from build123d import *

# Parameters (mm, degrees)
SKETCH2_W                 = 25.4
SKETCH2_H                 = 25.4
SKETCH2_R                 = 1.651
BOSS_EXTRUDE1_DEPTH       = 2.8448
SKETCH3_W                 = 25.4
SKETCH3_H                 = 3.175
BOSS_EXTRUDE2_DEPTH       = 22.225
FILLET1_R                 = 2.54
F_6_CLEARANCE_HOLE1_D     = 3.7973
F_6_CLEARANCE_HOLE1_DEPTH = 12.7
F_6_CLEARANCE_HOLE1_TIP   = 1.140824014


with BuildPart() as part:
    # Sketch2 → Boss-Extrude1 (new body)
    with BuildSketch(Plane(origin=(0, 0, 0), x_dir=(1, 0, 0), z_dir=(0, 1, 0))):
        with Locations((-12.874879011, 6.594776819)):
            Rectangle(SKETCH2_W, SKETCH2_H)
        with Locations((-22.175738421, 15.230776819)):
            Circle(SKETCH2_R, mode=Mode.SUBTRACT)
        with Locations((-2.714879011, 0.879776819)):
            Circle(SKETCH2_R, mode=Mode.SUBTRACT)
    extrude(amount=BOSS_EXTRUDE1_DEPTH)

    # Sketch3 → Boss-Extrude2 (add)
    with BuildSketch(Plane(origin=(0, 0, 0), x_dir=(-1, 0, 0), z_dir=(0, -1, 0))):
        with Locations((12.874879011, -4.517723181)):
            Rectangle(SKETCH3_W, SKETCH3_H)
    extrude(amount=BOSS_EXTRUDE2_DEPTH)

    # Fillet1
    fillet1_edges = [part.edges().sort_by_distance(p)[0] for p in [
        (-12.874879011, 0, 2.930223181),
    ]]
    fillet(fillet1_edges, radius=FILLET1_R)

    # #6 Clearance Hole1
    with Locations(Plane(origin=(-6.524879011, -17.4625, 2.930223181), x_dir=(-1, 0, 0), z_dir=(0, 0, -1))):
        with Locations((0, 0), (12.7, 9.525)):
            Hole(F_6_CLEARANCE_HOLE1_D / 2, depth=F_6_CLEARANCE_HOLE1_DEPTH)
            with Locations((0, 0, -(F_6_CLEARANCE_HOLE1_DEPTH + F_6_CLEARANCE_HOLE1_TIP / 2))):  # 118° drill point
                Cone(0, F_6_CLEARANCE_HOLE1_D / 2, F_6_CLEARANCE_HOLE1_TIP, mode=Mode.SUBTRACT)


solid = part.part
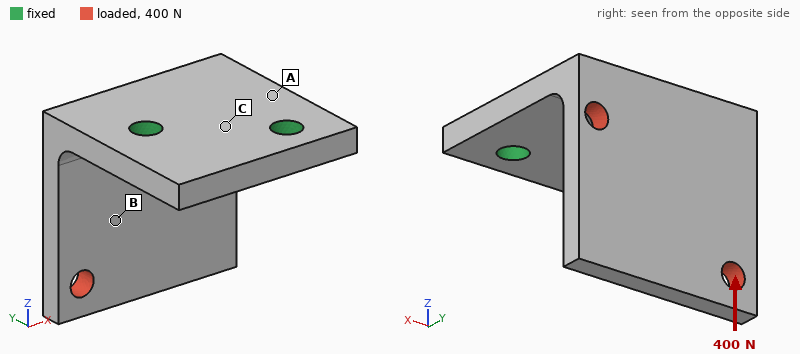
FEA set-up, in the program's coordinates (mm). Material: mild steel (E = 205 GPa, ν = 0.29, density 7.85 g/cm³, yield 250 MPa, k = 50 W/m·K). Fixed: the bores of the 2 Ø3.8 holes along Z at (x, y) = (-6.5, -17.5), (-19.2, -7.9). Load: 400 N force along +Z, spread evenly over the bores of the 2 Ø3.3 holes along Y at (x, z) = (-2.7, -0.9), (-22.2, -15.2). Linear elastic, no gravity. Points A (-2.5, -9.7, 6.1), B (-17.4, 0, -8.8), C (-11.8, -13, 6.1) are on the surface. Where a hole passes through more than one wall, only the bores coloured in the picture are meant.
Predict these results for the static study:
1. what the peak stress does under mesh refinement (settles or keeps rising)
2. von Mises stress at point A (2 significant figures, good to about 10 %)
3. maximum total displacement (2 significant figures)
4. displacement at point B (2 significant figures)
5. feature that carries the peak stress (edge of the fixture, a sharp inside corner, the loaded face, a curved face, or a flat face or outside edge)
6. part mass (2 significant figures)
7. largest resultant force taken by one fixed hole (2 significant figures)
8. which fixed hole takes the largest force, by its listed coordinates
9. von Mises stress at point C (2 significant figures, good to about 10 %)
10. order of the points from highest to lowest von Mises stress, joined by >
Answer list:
keeps rising
43 MPa
52 µm
25 µm
edge of the fixture
28 g
360 N
(-19.2, -7.9)
29 MPa
A > C > B
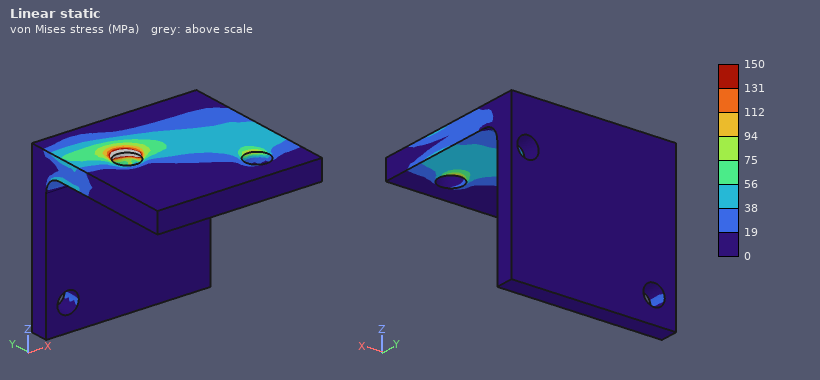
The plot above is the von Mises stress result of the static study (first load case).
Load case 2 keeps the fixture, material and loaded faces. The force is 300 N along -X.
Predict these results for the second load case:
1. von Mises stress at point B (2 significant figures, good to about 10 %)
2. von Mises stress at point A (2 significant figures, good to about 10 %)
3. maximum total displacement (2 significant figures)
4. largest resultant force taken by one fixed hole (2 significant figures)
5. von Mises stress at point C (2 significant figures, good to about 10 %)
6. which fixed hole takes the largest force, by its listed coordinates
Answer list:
9.9 MPa
38 MPa
39 µm
360 N
26 MPa
(-19.2, -7.9)
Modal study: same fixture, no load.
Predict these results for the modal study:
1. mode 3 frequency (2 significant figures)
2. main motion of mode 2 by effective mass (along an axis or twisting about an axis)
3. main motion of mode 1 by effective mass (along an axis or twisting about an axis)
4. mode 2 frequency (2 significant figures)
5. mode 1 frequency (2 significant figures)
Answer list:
9000 Hz
along X
along Y
4800 Hz
2900 Hz
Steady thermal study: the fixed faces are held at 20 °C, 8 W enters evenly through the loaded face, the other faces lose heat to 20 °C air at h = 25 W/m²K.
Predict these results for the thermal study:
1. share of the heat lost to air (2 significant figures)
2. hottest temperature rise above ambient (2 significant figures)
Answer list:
17 %
55 K
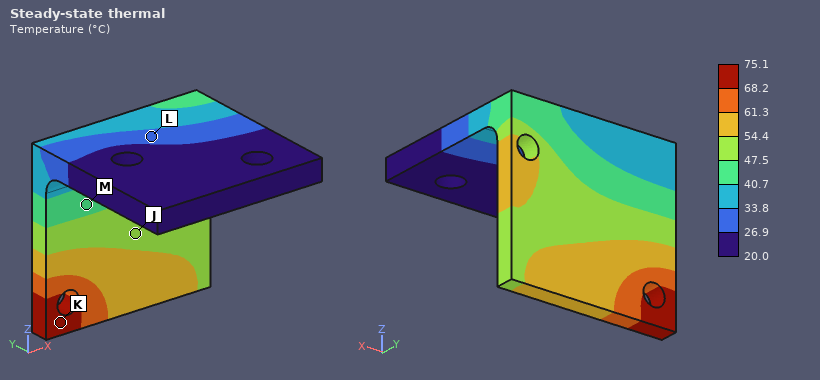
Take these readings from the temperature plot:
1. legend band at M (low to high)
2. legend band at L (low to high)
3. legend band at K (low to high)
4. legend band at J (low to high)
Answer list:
40.7 to 47.5 °C
26.9 to 33.8 °C
68.2 to 75.1 °C
47.5 to 54.4 °C
